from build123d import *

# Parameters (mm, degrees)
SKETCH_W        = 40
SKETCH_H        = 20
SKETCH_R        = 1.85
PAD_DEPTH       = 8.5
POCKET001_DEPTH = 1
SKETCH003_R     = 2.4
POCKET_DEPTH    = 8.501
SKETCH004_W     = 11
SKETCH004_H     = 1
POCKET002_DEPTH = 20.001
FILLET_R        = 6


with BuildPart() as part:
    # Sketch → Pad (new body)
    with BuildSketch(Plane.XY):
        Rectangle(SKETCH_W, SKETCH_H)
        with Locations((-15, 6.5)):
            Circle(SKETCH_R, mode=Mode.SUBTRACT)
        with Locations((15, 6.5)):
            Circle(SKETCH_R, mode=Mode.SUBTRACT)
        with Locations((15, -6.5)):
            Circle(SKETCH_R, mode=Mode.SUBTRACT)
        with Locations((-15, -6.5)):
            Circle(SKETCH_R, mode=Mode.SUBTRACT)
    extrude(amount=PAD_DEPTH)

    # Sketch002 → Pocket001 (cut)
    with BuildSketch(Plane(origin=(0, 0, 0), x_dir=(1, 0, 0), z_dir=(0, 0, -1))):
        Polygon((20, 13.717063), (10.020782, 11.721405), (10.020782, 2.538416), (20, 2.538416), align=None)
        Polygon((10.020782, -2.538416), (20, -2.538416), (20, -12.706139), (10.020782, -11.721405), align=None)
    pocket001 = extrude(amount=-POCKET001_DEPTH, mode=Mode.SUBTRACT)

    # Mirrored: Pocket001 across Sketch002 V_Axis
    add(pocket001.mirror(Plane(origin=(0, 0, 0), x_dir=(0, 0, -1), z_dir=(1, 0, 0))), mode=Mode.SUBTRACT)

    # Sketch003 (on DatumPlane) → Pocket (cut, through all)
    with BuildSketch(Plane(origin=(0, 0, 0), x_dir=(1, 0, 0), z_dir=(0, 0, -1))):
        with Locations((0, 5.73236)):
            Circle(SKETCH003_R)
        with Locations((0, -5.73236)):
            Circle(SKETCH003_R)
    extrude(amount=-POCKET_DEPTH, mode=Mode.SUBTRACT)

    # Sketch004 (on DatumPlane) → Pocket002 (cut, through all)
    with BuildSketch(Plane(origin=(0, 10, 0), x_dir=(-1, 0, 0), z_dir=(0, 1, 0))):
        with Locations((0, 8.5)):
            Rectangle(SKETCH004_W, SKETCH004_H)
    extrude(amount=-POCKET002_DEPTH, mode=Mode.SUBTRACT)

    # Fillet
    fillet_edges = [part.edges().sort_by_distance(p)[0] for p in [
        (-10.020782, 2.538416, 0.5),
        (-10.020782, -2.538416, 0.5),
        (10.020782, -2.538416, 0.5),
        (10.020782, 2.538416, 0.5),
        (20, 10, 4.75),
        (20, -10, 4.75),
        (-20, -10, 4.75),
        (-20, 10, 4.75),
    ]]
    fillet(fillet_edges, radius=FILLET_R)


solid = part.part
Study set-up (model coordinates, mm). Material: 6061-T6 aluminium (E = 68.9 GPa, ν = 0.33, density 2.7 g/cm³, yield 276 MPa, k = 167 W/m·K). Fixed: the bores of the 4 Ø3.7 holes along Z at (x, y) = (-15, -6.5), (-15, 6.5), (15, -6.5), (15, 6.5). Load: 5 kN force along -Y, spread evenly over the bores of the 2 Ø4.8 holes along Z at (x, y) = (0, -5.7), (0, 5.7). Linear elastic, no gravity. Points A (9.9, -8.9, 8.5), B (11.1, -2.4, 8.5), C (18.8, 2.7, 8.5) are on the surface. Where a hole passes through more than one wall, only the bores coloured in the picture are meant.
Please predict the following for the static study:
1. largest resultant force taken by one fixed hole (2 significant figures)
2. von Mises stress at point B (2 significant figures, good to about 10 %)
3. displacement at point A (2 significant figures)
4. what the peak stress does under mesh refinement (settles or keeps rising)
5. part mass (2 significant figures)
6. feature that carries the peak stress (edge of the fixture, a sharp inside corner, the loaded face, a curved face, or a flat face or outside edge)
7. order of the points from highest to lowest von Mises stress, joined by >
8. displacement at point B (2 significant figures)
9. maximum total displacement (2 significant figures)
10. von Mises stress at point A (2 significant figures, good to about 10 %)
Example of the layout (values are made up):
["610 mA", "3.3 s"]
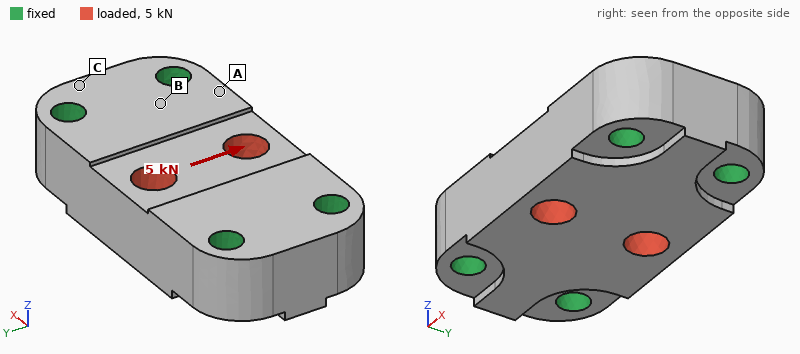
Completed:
["1.7 kN", "33 MPa", "3.8 µm", "keeps rising", "15 g", "edge of the fixture", "B > A > C", "2.2 µm", "13 µm", "13 MPa"]
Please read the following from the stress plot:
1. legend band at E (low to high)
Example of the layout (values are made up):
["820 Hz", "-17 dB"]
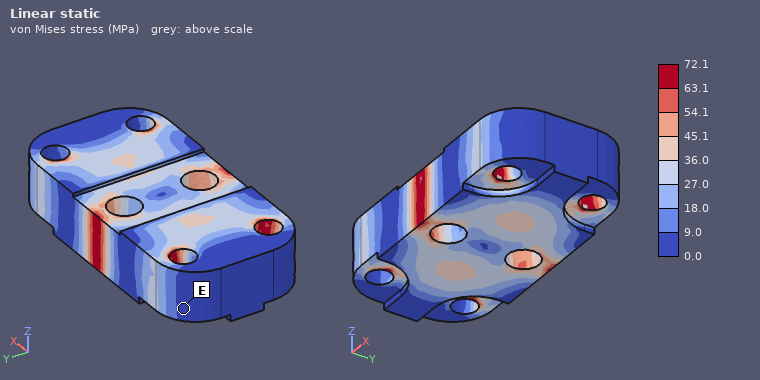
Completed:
["0.0 to 9.0 MPa"]
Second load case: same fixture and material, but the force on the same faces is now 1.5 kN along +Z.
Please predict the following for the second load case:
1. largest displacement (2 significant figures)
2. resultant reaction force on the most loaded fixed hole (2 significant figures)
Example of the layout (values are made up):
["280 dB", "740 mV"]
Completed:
["7.7 µm", "390 N"]
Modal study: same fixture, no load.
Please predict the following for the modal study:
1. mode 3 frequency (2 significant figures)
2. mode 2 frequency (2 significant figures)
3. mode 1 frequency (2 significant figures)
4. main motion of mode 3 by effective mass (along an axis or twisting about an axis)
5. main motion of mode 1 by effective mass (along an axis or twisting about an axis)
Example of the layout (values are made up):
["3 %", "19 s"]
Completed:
["49 kHz", "46 kHz", "34 kHz", "along Y", "along Z"]
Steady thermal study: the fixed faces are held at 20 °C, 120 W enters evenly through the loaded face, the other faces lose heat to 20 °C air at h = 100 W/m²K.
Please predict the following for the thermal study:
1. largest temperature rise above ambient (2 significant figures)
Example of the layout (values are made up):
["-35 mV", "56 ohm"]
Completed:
["32 K"]
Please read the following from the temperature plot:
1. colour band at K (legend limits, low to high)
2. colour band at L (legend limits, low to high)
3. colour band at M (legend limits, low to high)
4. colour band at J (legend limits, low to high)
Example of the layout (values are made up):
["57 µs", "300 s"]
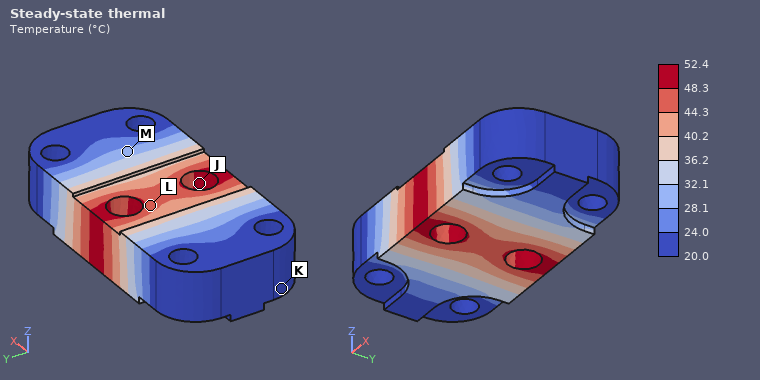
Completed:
["20.0 to 24.0 °C", "44.3 to 48.3 °C", "28.1 to 32.1 °C", "48.3 to 52.4 °C"]
